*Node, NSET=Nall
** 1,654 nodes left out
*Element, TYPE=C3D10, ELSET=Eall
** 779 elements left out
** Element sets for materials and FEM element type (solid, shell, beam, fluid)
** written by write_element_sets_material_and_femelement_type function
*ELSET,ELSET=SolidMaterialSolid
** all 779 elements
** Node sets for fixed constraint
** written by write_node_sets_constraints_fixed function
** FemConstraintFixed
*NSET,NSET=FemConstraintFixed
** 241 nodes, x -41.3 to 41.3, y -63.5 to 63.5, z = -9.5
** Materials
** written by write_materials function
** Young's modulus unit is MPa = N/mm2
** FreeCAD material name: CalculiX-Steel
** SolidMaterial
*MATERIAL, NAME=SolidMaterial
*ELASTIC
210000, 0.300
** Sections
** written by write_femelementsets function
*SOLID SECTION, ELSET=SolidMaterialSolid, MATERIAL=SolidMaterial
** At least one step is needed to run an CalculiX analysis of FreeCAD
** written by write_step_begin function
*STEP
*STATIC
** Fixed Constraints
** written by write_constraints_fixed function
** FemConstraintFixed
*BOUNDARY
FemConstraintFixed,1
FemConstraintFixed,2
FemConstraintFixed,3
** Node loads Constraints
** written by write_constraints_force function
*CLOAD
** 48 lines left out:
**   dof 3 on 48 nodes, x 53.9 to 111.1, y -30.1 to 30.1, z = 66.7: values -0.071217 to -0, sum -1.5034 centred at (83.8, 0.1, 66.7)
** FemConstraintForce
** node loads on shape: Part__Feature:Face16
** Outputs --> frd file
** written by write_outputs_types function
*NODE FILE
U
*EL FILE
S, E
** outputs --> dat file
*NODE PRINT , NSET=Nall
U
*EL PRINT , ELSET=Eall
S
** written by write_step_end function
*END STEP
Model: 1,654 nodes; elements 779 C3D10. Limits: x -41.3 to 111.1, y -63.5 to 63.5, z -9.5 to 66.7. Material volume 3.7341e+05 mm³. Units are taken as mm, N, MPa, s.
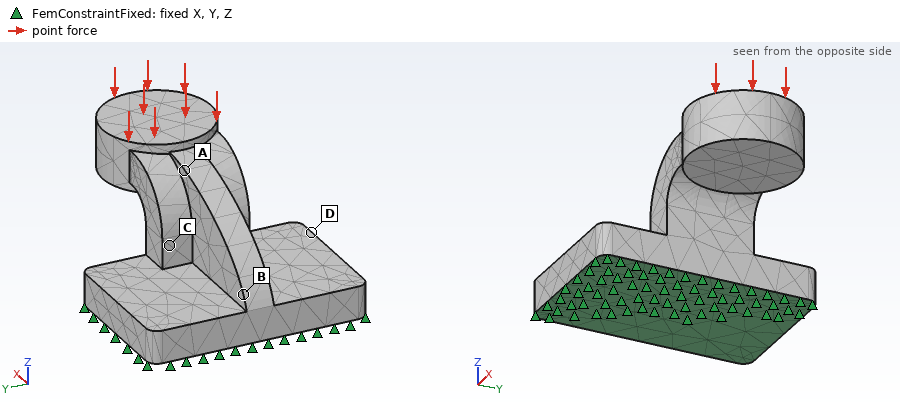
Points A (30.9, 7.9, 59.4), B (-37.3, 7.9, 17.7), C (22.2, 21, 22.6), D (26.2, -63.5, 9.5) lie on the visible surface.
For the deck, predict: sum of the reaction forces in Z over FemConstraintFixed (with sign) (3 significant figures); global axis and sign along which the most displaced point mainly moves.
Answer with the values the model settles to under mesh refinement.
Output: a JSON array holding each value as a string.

["1.50 N", "-Z"]
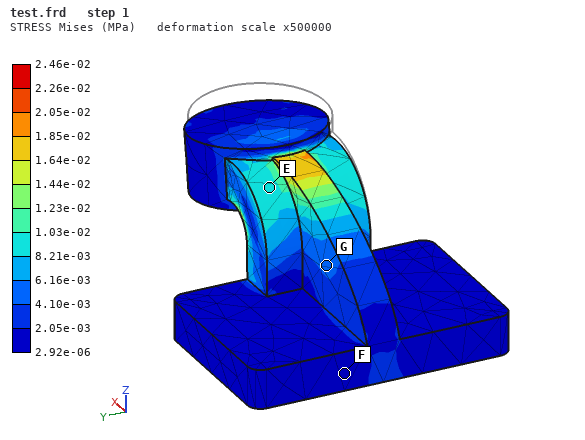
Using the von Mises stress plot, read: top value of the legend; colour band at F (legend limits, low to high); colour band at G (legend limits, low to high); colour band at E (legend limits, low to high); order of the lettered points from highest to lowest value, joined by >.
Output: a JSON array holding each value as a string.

["2.46e-02 MPa", "2.92e-06 to 2.05e-03 MPa", "4.10e-03 to 6.16e-03 MPa", "8.21e-03 to 1.03e-02 MPa", "E > G > F"]
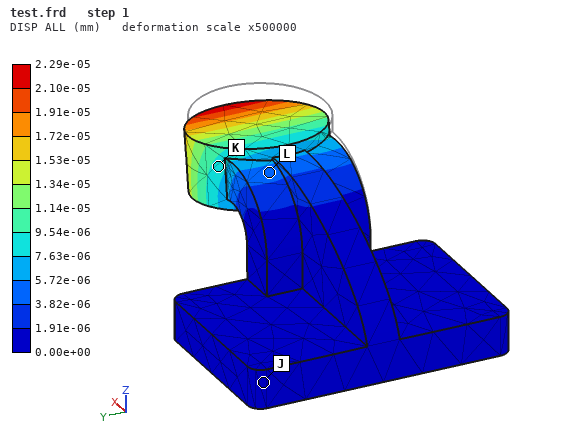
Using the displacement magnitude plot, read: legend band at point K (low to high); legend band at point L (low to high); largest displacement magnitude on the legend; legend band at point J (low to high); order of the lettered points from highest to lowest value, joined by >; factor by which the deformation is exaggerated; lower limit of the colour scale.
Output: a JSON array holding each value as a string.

["7.63e-06 to 9.54e-06 mm", "3.82e-06 to 5.72e-06 mm", "2.29e-05 mm", "0.00e+00 to 1.91e-06 mm", "K > L > J", "500000", "0.00e+00 mm"]
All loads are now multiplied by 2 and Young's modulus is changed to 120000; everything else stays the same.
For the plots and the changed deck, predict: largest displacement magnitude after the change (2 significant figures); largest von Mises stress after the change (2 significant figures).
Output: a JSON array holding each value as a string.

["8.0e-05 mm", "0.049 MPa"]
